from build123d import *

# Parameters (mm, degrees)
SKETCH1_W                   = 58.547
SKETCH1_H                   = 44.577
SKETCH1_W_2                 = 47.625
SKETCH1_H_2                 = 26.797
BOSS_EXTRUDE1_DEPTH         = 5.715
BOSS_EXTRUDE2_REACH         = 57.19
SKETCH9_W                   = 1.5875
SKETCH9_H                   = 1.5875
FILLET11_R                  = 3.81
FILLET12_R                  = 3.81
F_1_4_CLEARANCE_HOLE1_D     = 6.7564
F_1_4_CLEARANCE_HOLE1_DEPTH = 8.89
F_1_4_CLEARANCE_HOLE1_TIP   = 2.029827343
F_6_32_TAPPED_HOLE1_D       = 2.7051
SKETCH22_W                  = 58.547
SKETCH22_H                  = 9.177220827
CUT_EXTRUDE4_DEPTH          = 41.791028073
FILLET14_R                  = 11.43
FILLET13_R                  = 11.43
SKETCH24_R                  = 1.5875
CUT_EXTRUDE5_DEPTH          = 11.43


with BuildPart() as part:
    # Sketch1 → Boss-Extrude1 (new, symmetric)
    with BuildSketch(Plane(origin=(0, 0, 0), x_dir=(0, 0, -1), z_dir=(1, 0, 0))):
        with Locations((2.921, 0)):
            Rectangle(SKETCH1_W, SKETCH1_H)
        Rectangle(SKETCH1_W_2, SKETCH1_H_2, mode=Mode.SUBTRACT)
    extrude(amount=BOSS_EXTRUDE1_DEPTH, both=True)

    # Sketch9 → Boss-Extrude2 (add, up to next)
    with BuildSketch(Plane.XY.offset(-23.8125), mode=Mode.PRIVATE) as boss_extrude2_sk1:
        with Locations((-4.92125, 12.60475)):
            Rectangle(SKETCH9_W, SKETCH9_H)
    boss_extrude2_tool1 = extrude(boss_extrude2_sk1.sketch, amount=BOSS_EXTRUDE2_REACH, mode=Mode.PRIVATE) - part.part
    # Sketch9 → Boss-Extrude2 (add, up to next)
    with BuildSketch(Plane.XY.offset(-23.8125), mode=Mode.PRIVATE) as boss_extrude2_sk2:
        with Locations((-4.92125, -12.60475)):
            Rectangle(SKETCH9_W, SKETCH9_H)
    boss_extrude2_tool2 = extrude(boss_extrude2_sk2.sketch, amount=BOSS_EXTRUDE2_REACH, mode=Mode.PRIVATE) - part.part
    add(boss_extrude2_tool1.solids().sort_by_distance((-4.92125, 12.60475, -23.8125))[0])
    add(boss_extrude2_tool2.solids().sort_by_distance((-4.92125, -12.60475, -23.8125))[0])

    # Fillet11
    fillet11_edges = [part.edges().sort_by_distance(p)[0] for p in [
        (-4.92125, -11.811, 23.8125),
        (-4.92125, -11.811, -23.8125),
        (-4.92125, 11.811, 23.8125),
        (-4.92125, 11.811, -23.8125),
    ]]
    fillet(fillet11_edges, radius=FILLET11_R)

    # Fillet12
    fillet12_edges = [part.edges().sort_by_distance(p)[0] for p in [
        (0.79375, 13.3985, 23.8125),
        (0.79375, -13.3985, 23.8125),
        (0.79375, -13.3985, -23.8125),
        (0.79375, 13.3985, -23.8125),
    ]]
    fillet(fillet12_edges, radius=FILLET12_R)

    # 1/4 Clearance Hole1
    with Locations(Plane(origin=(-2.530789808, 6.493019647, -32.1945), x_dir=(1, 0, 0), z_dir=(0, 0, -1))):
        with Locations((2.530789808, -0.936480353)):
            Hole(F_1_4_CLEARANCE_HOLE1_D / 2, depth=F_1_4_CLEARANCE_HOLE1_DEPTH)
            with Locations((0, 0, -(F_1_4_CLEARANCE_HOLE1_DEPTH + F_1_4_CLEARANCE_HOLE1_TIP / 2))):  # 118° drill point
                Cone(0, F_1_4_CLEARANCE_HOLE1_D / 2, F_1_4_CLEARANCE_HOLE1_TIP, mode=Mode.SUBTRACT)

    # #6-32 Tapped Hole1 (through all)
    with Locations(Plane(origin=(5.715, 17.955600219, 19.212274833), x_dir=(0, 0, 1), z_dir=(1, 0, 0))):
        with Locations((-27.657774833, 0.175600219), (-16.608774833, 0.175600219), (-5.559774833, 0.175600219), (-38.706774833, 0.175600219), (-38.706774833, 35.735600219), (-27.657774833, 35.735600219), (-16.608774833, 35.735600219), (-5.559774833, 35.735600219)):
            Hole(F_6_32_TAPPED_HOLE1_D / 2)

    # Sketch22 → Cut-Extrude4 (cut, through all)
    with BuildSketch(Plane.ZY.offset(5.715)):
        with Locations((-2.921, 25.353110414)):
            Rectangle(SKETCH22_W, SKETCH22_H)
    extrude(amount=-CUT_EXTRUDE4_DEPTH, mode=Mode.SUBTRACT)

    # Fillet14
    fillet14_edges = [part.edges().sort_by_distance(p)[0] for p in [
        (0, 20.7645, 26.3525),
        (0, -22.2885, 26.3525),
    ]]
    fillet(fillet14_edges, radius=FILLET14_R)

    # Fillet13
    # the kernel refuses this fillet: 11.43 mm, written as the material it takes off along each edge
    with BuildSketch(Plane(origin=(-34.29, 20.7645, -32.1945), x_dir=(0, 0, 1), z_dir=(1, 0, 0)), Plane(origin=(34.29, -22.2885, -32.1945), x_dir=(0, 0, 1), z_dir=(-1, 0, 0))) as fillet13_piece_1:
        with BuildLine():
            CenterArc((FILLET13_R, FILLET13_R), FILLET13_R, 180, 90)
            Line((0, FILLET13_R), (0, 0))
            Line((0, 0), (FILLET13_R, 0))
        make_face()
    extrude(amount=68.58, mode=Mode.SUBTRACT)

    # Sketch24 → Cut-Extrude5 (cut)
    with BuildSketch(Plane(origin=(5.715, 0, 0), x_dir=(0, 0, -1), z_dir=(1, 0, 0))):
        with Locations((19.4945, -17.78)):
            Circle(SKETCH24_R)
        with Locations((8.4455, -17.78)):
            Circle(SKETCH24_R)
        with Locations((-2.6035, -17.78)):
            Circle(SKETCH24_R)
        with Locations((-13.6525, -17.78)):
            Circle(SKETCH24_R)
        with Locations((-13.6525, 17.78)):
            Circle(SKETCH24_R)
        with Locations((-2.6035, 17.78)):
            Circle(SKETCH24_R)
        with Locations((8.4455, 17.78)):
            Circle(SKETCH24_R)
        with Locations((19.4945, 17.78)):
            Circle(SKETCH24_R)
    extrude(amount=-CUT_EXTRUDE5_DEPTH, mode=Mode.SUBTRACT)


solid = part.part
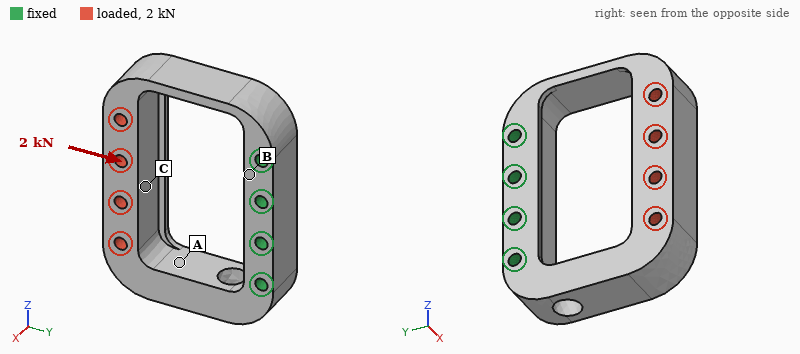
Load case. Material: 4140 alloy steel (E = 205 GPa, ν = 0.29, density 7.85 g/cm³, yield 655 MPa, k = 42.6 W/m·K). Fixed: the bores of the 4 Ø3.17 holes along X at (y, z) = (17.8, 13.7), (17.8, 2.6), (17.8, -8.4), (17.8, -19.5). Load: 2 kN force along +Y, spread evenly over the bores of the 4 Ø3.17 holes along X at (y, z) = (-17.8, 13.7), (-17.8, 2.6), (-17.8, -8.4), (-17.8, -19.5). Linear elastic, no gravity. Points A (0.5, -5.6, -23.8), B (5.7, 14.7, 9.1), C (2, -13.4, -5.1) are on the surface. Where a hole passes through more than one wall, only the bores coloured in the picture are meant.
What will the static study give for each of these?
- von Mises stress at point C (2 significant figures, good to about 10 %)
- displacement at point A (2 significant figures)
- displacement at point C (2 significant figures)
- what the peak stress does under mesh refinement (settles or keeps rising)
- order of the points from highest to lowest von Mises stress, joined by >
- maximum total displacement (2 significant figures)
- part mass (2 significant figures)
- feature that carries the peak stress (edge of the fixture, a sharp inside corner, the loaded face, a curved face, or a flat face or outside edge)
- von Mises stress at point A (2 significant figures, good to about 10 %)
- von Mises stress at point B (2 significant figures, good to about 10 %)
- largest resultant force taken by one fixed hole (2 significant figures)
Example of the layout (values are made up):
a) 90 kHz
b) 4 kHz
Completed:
a) 74 MPa
b) 11 µm
c) 39 µm
d) keeps rising
e) C > A > B
f) 42 µm
g) 97 g
h) a sharp inside corner
i) 49 MPa
j) 15 MPa
k) 1.3 kN
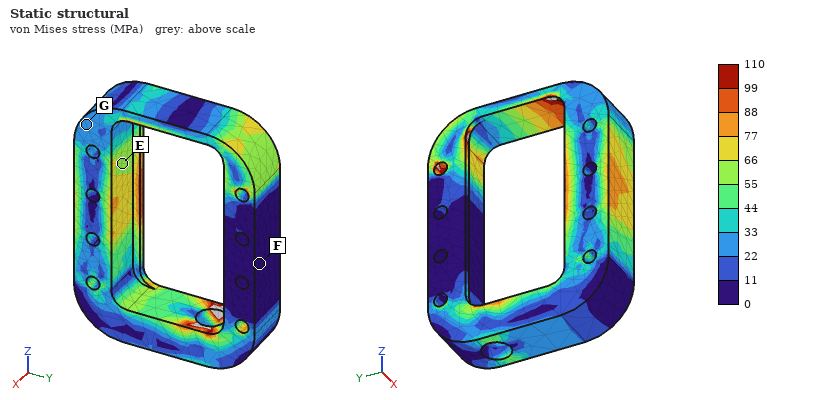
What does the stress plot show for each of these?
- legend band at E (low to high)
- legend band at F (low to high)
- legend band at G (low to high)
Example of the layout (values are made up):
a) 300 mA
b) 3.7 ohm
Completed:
a) 55 to 66 MPa
b) 0 to 11 MPa
c) 22 to 33 MPa
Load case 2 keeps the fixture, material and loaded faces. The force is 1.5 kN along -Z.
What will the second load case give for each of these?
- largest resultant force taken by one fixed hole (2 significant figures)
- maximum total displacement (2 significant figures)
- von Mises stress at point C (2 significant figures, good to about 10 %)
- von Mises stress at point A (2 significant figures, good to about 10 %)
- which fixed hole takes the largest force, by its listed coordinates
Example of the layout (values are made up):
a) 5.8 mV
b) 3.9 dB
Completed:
a) 1.4 kN
b) 0.13 mm
c) 74 MPa
d) 62 MPa
e) (17.8, -19.5)
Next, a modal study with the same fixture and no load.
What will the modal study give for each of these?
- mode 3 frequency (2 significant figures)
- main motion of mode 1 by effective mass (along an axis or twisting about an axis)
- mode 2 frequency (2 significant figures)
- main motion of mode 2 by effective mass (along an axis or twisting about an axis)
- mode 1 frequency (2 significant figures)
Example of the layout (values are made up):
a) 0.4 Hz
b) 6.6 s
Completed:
a) 4900 Hz
b) along X
c) 2500 Hz
d) along Z
e) 2100 Hz
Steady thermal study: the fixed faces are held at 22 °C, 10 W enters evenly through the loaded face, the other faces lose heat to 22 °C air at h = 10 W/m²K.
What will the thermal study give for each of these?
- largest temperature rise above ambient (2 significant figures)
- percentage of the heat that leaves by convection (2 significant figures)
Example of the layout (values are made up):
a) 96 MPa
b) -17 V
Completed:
a) 80 K
b) 24 %
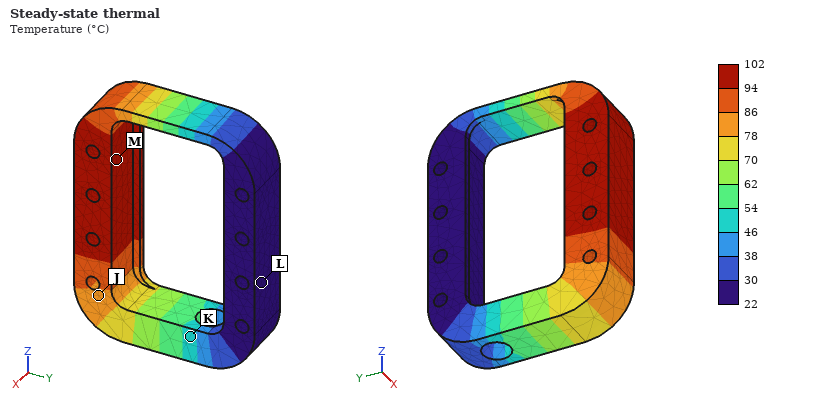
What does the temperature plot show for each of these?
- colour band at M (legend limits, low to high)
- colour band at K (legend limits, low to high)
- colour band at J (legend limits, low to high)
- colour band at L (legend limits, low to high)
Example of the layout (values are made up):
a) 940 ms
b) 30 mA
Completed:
a) 94 to 102 °C
b) 46 to 54 °C
c) 78 to 86 °C
d) 22 to 30 °C
